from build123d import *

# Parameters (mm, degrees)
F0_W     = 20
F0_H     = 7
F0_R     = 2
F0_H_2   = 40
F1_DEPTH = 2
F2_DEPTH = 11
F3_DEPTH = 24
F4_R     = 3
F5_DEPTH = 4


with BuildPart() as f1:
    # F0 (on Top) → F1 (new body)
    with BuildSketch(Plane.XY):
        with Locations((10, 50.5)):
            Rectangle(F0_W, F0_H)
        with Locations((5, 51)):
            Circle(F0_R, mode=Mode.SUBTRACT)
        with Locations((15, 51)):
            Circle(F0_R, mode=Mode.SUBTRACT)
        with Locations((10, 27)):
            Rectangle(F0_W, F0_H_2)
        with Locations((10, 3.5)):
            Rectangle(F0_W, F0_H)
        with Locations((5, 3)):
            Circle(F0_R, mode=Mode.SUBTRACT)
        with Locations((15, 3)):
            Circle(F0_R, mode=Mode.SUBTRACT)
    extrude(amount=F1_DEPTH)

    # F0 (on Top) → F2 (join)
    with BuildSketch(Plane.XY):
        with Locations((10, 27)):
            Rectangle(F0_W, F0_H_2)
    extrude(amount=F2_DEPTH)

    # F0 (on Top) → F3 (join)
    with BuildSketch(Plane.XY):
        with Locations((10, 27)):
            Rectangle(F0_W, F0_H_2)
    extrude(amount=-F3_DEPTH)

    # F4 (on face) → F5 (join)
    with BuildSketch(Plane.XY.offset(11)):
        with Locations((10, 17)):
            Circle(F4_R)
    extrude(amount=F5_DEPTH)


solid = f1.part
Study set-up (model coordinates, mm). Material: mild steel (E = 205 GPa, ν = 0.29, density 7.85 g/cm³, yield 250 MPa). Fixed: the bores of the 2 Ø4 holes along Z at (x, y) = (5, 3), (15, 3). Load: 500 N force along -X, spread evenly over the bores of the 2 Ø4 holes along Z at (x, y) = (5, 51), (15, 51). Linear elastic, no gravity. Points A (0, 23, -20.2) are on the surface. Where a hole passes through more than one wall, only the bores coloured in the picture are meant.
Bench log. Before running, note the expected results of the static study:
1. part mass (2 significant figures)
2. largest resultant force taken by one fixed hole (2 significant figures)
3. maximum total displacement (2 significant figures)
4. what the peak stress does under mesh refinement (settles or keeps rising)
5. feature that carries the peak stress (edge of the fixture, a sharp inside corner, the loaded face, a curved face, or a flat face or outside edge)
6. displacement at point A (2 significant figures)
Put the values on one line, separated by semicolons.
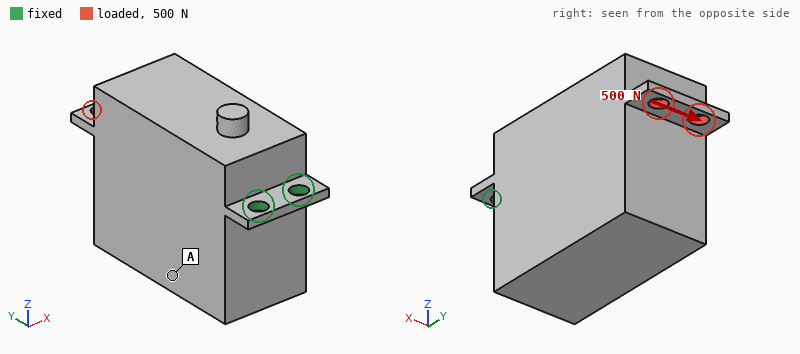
220 g; 1.9 kN; 35 µm; keeps rising; edge of the fixture; 13 µm
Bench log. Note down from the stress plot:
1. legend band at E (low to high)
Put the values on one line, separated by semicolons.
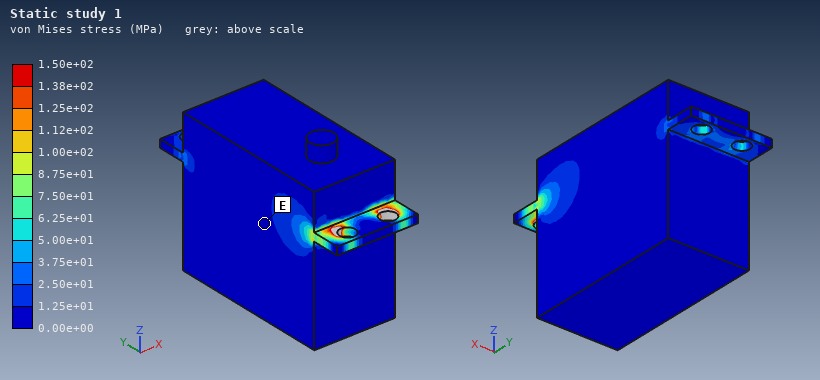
0.00e+00 to 1.25e+01 MPa
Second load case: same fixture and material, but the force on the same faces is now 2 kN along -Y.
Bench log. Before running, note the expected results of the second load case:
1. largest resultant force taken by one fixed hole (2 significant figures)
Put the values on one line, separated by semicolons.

1.0 kN
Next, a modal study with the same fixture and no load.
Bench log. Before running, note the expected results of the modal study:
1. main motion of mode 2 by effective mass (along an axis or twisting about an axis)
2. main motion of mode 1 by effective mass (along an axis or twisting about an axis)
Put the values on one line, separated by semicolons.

along X; along Z
